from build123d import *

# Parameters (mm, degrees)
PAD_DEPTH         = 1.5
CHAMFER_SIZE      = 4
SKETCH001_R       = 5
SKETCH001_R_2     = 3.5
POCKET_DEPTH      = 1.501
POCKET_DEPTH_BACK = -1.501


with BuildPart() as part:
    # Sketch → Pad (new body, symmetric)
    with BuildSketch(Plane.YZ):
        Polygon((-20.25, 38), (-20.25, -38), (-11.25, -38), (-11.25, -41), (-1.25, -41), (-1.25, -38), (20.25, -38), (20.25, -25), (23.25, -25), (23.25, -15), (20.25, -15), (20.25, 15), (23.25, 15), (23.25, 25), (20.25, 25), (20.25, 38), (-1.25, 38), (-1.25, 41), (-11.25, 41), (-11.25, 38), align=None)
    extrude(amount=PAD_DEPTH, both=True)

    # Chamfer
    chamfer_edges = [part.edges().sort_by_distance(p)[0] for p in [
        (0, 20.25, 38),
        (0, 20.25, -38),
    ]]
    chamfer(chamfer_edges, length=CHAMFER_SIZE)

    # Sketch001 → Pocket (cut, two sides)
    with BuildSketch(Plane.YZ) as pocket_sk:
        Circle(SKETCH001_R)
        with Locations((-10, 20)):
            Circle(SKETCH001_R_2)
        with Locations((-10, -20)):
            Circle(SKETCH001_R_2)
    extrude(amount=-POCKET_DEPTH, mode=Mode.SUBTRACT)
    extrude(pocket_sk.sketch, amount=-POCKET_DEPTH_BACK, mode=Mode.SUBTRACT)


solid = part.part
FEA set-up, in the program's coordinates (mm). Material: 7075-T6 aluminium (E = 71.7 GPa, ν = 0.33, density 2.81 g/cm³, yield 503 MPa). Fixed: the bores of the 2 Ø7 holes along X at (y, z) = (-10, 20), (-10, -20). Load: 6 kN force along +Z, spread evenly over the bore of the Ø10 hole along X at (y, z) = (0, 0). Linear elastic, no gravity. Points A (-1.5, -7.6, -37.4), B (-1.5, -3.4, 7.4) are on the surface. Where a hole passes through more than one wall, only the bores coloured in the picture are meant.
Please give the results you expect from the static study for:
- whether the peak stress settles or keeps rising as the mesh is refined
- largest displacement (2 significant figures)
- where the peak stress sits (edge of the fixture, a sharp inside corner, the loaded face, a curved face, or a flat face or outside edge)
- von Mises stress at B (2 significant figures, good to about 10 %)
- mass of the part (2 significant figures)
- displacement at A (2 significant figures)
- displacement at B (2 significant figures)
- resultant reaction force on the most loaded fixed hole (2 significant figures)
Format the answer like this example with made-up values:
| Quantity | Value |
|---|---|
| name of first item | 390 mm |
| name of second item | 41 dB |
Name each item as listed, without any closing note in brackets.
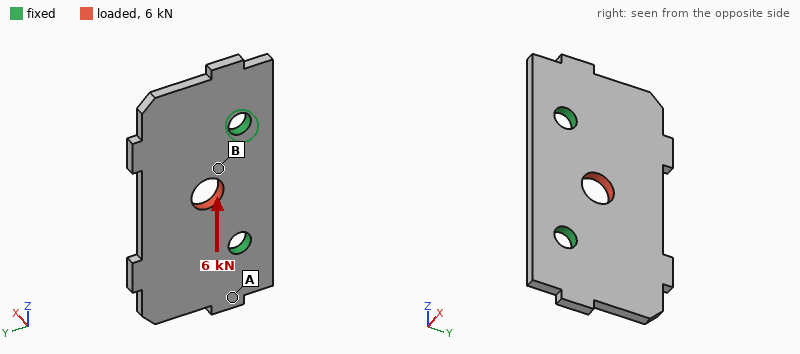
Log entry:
| Quantity | Value |
|---|---|
| whether the peak stress settles or keeps rising as the mesh is refined | keeps rising |
| largest displacement | 28 µm |
| where the peak stress sits | edge of the fixture |
| von Mises stress at B | 69 MPa |
| mass of the part | 26 g |
| displacement at A | 12 µm |
| displacement at B | 13 µm |
| resultant reaction force on the most loaded fixed hole | 3.2 kN |
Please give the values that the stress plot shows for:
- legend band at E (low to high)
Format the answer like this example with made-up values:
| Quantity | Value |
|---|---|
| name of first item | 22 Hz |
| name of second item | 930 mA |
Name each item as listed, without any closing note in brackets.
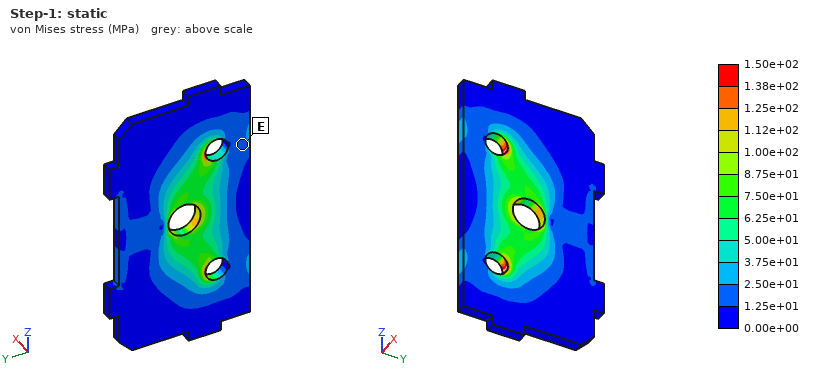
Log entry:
| Quantity | Value |
|---|---|
| legend band at E | 1.25e+01 to 2.50e+01 MPa |
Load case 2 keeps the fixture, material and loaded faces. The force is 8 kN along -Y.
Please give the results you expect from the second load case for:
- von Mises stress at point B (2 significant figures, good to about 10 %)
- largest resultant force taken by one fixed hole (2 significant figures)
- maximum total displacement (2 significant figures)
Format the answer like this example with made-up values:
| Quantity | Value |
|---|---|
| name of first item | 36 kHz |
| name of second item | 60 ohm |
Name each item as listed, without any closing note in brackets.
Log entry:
| Quantity | Value |
|---|---|
| von Mises stress at point B | 79 MPa |
| largest resultant force taken by one fixed hole | 4.2 kN |
| maximum total displacement | 36 µm |
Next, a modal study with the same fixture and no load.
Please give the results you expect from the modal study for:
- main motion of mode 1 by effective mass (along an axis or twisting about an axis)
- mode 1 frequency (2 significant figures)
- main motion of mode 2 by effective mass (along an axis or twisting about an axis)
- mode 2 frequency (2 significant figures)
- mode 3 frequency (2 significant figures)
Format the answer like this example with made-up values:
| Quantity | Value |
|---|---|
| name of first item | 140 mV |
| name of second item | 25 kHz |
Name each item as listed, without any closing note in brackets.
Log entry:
| Quantity | Value |
|---|---|
| main motion of mode 1 by effective mass | along X |
| mode 1 frequency | 2600 Hz |
| main motion of mode 2 by effective mass | twisting about Y |
| mode 2 frequency | 3500 Hz |
| mode 3 frequency | 5100 Hz |
